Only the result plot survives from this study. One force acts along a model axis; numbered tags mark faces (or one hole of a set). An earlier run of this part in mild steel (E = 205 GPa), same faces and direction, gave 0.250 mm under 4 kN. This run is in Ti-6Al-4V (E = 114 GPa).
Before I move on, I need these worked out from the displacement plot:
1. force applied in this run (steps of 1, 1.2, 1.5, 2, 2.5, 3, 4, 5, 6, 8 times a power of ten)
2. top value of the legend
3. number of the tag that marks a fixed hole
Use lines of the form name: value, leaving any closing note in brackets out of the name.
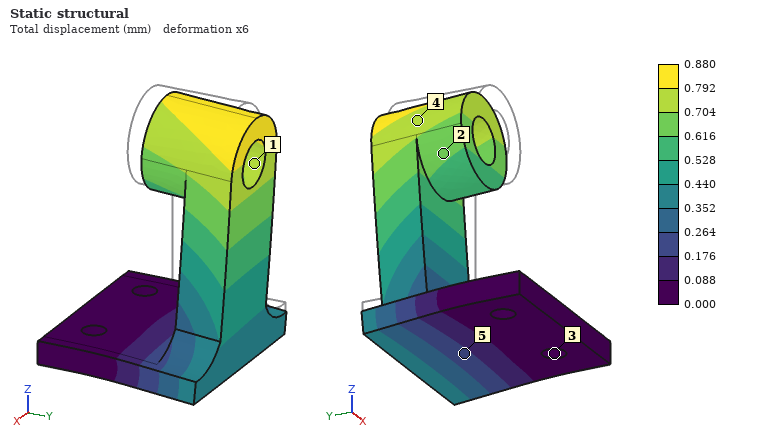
force applied in this run: 8 kN
top value of the legend: 0.880 mm
number of the tag that marks a fixed hole: 3
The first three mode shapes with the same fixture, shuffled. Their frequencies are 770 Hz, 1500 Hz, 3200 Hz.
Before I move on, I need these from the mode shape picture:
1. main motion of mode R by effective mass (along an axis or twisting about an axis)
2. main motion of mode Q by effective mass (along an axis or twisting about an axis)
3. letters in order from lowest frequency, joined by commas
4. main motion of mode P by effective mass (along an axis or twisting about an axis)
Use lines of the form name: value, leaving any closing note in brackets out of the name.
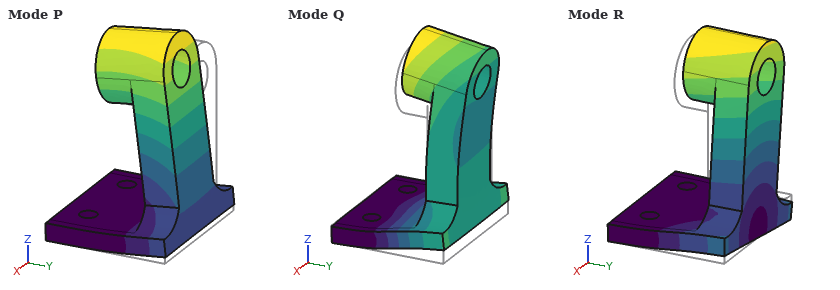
main motion of mode R by effective mass: along X
main motion of mode Q by effective mass: along Z
letters in order from lowest frequency, joined by commas: P, R, Q
main motion of mode P by effective mass: along Y
